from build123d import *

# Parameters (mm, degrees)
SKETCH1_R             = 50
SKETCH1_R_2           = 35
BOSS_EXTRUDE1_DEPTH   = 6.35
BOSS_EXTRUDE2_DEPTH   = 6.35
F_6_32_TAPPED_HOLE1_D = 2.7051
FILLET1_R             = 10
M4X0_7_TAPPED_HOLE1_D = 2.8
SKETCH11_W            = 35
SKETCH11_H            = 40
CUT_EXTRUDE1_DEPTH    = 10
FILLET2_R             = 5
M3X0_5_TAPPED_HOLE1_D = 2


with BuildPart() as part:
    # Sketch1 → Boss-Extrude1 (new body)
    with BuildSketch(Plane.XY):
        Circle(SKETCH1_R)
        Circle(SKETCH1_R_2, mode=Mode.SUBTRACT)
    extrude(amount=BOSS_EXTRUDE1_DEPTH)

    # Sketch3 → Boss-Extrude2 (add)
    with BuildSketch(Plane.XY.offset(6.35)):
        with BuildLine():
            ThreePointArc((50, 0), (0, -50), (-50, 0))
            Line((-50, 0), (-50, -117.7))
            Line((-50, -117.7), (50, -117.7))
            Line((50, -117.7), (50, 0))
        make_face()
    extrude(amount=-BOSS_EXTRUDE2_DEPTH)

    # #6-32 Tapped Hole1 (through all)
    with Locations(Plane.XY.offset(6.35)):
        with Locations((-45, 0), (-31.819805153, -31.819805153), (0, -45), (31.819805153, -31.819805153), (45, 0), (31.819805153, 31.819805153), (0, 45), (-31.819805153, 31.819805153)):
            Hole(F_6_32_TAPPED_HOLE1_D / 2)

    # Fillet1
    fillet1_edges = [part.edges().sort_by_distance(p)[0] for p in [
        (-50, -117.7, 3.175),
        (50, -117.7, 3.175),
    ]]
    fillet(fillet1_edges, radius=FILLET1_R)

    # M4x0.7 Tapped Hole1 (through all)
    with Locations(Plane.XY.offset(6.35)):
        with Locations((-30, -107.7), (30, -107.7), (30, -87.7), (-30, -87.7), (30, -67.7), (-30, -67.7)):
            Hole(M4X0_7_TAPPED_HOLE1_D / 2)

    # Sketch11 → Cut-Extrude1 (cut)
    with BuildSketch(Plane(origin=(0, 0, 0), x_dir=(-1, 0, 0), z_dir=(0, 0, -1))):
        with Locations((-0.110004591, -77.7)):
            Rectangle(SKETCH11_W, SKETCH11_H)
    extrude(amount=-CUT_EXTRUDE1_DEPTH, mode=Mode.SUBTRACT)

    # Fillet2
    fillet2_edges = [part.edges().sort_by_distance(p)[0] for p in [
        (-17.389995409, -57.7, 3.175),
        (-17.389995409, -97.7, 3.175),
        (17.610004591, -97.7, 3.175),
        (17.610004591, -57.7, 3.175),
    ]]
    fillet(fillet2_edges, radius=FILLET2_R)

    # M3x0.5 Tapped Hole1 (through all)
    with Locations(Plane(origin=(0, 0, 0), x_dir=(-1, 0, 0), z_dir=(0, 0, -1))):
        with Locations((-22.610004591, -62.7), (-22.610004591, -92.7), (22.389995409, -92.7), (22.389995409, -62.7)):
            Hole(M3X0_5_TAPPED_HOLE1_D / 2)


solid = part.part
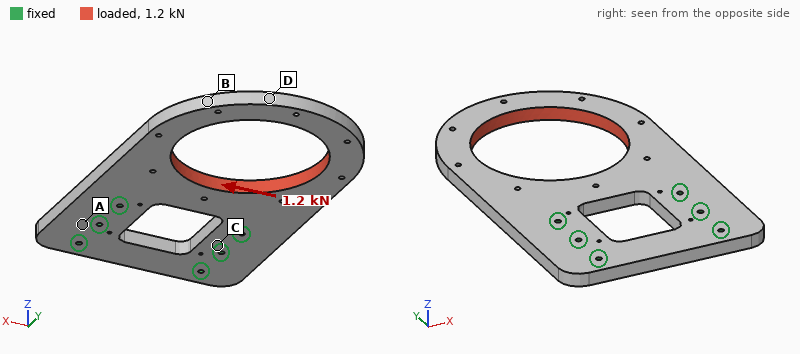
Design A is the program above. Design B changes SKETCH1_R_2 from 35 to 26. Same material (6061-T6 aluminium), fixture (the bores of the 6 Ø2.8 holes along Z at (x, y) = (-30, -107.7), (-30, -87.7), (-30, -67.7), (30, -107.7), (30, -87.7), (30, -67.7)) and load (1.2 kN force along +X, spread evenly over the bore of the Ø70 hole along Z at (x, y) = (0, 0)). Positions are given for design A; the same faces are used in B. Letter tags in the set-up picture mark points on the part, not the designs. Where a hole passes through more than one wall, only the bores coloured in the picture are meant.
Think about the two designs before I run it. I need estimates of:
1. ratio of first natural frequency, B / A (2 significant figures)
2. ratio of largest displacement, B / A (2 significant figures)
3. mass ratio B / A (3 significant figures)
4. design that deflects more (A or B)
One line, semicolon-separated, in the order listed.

0.94; 0.44; 1.17; A
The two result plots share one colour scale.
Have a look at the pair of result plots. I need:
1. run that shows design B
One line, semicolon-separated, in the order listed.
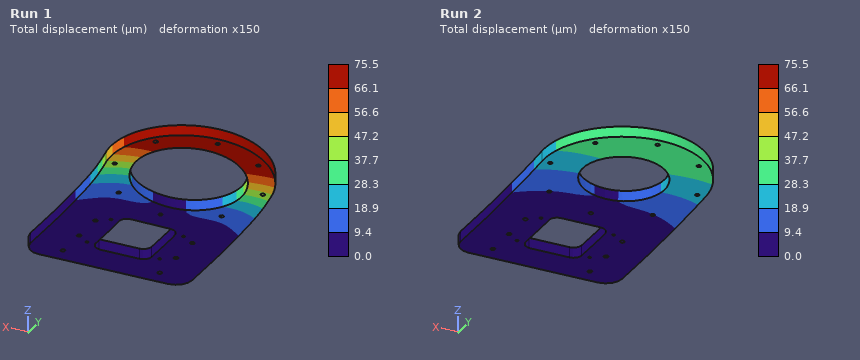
Run 2
